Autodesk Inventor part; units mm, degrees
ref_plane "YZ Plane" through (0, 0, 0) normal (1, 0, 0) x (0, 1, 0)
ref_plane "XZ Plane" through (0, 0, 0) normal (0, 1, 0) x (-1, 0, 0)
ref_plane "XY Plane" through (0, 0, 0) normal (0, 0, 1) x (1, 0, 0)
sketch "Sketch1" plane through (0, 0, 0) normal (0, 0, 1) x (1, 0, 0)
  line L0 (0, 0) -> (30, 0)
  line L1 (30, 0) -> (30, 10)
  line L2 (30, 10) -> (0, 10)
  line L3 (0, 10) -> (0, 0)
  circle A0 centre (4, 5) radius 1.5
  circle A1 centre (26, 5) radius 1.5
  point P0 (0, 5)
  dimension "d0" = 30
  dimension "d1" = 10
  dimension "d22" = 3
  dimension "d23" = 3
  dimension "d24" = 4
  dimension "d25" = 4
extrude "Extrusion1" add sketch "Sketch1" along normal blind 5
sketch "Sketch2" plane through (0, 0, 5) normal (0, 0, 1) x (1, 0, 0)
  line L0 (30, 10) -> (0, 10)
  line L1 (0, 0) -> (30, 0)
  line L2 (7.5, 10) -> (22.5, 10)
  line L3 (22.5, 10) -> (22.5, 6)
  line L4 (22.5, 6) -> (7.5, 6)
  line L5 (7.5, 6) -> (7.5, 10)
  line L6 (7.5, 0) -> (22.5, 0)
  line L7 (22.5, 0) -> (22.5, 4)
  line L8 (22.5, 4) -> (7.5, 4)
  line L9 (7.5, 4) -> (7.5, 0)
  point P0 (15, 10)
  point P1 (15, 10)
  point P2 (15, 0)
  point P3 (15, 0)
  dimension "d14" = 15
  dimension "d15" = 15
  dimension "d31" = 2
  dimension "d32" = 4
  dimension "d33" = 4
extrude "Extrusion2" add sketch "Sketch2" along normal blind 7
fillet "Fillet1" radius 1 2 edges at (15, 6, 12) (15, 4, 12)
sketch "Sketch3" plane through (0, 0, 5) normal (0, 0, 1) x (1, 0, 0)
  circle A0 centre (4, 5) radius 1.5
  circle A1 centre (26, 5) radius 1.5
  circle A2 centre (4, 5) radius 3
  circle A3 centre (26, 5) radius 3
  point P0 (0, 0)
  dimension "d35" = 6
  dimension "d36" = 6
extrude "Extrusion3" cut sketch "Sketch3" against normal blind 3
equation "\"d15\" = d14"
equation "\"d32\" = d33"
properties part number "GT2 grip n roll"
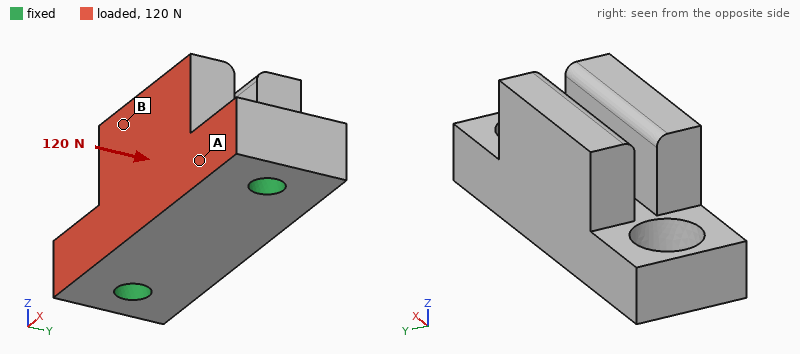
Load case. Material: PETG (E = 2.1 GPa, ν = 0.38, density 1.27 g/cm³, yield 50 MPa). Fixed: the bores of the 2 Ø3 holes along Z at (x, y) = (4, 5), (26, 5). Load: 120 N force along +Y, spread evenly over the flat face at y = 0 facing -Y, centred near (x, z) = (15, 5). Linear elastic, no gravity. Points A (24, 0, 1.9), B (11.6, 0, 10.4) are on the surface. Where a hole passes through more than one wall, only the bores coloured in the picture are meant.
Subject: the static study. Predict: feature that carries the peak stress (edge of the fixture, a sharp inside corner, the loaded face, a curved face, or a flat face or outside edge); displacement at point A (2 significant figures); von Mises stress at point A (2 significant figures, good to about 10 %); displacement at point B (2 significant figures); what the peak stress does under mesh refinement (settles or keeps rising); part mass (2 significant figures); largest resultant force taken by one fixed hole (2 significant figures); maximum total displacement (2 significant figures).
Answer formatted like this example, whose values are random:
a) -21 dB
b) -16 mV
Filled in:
a) edge of the fixture
b) 0.062 mm
c) 4.4 MPa
d) 0.19 mm
e) keeps rising
f) 2.7 g
g) 60 N
h) 0.22 mm
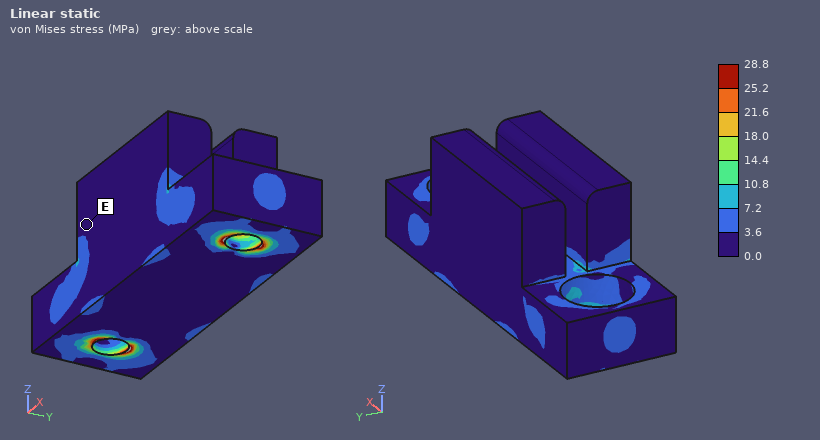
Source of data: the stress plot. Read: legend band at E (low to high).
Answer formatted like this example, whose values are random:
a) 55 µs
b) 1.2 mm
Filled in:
a) 0.0 to 3.6 MPa
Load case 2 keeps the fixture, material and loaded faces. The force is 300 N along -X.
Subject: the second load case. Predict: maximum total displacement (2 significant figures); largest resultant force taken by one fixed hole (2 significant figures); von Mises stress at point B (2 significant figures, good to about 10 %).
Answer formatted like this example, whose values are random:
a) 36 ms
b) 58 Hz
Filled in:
a) 78 µm
b) 170 N
c) 3.7 MPa
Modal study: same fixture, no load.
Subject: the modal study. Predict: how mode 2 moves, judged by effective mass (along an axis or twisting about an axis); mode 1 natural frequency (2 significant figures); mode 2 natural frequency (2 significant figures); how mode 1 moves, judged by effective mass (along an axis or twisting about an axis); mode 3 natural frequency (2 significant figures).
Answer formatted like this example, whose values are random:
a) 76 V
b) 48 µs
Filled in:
a) along Z
b) 2900 Hz
c) 7200 Hz
d) along Y
e) 9100 Hz
